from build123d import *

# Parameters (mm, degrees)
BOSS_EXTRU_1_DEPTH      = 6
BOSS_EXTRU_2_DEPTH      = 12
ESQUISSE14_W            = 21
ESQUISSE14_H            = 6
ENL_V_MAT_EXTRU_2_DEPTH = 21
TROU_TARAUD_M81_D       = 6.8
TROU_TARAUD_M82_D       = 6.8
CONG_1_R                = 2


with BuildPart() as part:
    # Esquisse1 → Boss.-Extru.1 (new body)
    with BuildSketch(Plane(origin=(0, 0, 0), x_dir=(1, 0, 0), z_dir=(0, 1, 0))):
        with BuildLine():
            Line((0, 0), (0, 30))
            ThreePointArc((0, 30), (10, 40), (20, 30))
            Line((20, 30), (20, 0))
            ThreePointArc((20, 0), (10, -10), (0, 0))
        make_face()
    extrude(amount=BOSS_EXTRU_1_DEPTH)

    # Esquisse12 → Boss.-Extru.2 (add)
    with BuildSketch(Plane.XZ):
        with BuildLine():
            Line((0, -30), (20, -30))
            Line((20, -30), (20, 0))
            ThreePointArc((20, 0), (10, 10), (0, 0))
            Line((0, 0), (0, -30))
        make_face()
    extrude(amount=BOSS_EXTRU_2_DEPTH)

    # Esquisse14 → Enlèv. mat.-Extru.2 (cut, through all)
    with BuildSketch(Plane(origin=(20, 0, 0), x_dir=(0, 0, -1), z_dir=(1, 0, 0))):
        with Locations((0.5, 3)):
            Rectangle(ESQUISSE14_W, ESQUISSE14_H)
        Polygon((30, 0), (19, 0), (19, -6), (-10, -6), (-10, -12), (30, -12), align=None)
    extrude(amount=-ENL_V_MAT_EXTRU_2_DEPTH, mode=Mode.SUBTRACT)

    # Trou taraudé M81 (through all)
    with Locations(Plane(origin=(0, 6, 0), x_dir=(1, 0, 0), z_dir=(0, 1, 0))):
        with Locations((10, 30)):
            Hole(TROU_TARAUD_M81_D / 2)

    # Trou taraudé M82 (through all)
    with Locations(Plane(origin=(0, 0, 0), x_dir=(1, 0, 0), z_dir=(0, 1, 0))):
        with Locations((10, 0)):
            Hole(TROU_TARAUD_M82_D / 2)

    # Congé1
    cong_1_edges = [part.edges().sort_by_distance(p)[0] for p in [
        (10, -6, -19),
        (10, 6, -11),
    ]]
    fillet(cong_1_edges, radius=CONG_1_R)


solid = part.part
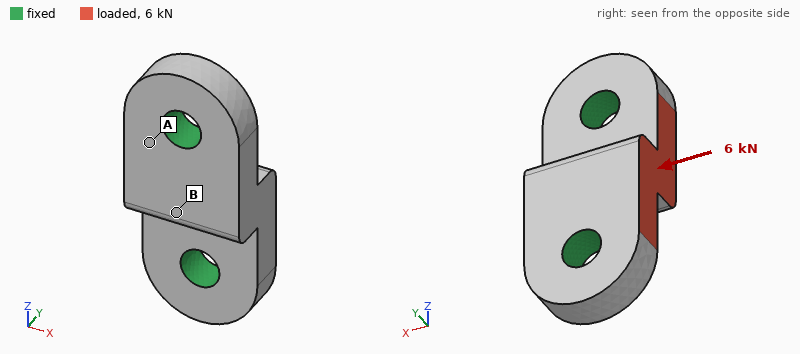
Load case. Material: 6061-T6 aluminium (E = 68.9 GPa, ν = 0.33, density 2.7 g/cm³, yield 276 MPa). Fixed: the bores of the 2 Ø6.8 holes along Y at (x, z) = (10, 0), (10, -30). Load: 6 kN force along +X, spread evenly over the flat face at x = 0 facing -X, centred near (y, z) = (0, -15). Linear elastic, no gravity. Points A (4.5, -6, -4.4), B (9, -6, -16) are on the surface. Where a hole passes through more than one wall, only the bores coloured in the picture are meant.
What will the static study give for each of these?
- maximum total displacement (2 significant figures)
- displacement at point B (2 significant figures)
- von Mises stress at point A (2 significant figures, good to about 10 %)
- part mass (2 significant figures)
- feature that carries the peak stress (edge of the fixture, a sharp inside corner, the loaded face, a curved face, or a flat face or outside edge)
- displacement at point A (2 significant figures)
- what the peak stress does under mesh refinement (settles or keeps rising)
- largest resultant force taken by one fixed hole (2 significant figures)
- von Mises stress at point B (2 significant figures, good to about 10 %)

16 µm
12 µm
47 MPa
16 g
edge of the fixture
5.3 µm
keeps rising
3.0 kN
20 MPa
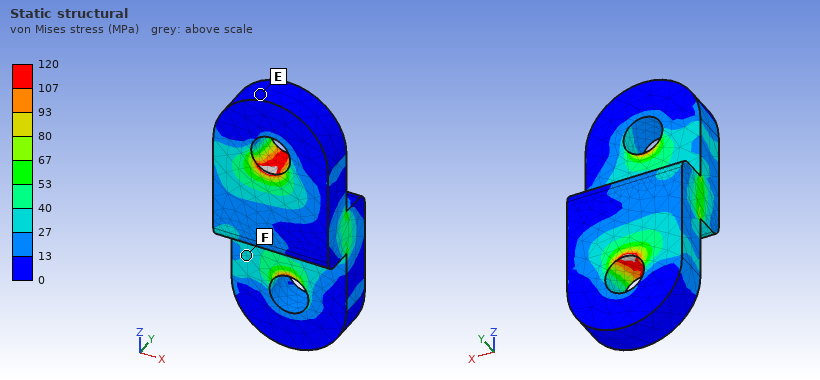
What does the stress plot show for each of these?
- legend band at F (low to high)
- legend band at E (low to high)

27 to 40 MPa
0 to 13 MPa
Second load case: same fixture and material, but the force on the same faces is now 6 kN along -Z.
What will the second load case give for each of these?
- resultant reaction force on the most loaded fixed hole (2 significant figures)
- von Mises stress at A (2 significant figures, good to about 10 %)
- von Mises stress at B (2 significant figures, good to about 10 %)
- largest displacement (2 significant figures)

3.3 kN
32 MPa
20 MPa
26 µm
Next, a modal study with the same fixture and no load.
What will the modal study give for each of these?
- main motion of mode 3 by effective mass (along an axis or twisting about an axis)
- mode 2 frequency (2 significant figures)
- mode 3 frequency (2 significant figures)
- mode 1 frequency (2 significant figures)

along X
26 kHz
34 kHz
26 kHz
